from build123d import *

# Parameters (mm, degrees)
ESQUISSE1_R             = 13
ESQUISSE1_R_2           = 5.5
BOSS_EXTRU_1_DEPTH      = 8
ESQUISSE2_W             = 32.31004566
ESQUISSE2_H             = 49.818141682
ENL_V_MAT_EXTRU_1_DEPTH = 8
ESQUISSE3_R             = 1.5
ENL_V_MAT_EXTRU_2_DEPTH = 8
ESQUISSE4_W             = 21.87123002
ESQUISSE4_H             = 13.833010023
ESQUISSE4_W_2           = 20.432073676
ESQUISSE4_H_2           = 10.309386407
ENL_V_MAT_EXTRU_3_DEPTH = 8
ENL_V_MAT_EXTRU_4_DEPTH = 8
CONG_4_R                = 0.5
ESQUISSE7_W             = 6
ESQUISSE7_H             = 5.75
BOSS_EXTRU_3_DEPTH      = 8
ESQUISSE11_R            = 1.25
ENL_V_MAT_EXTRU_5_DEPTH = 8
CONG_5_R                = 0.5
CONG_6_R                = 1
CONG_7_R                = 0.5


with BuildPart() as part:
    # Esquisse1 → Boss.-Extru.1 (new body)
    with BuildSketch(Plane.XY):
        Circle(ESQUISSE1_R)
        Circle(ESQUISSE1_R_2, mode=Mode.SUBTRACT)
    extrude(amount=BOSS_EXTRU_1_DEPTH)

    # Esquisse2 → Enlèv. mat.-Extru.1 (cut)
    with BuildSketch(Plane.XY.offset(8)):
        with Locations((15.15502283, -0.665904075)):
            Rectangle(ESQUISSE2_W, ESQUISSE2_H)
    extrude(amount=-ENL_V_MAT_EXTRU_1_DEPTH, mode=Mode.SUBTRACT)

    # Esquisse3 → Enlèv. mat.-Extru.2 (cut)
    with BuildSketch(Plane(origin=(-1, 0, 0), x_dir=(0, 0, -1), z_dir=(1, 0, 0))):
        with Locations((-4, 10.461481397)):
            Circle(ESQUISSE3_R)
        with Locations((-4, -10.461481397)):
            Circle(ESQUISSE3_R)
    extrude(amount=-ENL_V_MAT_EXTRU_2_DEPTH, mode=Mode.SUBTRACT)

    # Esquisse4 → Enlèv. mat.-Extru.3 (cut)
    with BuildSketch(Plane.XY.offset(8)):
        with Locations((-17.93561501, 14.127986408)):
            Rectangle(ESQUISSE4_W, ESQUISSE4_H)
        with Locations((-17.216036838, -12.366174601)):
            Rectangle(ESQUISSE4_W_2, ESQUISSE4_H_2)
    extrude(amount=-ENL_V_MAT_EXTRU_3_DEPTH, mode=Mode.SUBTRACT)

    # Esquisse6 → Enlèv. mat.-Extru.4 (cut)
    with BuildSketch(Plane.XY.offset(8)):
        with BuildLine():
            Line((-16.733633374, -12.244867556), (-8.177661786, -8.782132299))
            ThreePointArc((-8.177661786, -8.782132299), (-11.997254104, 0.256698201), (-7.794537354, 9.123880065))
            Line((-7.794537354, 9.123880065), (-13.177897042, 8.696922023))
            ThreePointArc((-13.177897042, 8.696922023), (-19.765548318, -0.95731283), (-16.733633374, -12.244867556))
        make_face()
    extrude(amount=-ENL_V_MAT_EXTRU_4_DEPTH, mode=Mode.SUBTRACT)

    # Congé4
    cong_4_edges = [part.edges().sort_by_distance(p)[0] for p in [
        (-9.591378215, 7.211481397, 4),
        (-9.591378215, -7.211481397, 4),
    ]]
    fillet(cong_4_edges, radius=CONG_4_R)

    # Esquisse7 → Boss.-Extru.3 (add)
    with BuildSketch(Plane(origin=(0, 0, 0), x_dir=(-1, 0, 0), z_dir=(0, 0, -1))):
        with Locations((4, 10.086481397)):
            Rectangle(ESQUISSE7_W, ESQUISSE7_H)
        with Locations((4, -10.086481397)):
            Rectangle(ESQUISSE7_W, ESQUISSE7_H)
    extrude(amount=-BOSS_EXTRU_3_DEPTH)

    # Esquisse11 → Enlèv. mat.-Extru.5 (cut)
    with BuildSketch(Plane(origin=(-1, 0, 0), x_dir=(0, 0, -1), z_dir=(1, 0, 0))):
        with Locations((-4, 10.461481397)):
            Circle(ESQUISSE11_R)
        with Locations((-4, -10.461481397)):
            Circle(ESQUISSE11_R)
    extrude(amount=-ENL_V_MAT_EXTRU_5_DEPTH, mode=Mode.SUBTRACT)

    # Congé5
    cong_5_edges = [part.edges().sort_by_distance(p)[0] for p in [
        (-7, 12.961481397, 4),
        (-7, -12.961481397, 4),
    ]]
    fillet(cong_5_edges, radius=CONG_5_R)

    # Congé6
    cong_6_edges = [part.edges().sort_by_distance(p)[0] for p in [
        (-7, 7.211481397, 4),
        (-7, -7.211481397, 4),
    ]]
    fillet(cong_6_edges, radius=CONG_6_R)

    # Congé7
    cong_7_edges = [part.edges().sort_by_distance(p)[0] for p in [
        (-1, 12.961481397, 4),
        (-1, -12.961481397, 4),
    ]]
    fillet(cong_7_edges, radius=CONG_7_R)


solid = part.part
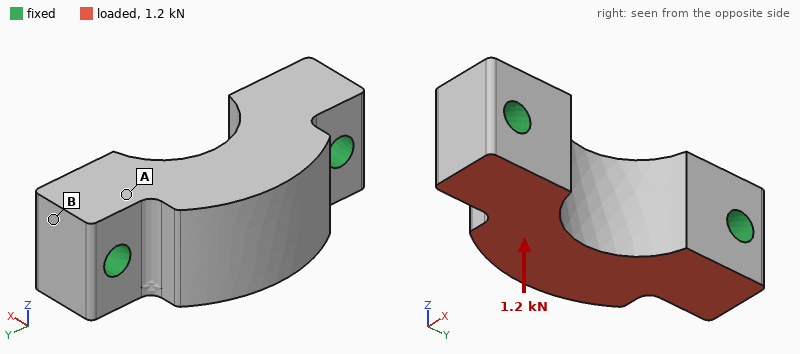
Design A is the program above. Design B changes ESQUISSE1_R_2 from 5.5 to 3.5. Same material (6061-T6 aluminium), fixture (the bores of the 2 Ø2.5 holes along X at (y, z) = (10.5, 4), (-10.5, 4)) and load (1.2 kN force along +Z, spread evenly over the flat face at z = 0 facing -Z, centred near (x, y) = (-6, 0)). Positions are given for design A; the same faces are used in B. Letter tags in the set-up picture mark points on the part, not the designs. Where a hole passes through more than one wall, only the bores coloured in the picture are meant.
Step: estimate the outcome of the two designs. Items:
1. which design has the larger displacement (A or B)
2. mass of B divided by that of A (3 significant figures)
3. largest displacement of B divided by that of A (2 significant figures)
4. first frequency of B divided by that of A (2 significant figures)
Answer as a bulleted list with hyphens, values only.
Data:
- A
- 1.14
- 0.86
- 1.0
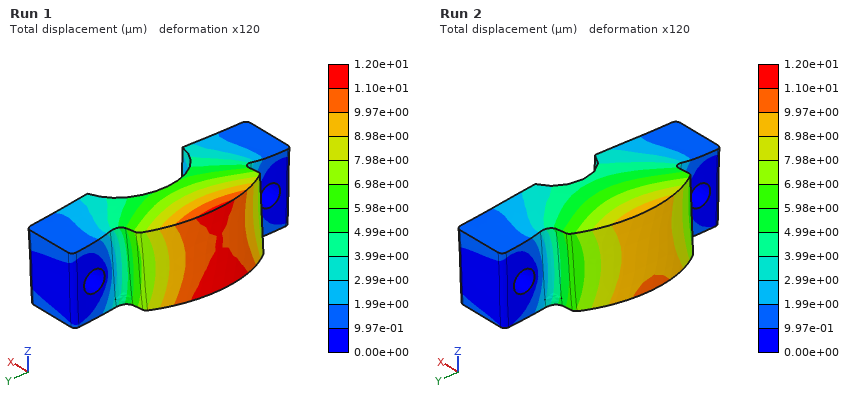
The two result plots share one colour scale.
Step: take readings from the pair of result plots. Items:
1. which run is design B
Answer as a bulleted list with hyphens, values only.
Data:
- Run 2
